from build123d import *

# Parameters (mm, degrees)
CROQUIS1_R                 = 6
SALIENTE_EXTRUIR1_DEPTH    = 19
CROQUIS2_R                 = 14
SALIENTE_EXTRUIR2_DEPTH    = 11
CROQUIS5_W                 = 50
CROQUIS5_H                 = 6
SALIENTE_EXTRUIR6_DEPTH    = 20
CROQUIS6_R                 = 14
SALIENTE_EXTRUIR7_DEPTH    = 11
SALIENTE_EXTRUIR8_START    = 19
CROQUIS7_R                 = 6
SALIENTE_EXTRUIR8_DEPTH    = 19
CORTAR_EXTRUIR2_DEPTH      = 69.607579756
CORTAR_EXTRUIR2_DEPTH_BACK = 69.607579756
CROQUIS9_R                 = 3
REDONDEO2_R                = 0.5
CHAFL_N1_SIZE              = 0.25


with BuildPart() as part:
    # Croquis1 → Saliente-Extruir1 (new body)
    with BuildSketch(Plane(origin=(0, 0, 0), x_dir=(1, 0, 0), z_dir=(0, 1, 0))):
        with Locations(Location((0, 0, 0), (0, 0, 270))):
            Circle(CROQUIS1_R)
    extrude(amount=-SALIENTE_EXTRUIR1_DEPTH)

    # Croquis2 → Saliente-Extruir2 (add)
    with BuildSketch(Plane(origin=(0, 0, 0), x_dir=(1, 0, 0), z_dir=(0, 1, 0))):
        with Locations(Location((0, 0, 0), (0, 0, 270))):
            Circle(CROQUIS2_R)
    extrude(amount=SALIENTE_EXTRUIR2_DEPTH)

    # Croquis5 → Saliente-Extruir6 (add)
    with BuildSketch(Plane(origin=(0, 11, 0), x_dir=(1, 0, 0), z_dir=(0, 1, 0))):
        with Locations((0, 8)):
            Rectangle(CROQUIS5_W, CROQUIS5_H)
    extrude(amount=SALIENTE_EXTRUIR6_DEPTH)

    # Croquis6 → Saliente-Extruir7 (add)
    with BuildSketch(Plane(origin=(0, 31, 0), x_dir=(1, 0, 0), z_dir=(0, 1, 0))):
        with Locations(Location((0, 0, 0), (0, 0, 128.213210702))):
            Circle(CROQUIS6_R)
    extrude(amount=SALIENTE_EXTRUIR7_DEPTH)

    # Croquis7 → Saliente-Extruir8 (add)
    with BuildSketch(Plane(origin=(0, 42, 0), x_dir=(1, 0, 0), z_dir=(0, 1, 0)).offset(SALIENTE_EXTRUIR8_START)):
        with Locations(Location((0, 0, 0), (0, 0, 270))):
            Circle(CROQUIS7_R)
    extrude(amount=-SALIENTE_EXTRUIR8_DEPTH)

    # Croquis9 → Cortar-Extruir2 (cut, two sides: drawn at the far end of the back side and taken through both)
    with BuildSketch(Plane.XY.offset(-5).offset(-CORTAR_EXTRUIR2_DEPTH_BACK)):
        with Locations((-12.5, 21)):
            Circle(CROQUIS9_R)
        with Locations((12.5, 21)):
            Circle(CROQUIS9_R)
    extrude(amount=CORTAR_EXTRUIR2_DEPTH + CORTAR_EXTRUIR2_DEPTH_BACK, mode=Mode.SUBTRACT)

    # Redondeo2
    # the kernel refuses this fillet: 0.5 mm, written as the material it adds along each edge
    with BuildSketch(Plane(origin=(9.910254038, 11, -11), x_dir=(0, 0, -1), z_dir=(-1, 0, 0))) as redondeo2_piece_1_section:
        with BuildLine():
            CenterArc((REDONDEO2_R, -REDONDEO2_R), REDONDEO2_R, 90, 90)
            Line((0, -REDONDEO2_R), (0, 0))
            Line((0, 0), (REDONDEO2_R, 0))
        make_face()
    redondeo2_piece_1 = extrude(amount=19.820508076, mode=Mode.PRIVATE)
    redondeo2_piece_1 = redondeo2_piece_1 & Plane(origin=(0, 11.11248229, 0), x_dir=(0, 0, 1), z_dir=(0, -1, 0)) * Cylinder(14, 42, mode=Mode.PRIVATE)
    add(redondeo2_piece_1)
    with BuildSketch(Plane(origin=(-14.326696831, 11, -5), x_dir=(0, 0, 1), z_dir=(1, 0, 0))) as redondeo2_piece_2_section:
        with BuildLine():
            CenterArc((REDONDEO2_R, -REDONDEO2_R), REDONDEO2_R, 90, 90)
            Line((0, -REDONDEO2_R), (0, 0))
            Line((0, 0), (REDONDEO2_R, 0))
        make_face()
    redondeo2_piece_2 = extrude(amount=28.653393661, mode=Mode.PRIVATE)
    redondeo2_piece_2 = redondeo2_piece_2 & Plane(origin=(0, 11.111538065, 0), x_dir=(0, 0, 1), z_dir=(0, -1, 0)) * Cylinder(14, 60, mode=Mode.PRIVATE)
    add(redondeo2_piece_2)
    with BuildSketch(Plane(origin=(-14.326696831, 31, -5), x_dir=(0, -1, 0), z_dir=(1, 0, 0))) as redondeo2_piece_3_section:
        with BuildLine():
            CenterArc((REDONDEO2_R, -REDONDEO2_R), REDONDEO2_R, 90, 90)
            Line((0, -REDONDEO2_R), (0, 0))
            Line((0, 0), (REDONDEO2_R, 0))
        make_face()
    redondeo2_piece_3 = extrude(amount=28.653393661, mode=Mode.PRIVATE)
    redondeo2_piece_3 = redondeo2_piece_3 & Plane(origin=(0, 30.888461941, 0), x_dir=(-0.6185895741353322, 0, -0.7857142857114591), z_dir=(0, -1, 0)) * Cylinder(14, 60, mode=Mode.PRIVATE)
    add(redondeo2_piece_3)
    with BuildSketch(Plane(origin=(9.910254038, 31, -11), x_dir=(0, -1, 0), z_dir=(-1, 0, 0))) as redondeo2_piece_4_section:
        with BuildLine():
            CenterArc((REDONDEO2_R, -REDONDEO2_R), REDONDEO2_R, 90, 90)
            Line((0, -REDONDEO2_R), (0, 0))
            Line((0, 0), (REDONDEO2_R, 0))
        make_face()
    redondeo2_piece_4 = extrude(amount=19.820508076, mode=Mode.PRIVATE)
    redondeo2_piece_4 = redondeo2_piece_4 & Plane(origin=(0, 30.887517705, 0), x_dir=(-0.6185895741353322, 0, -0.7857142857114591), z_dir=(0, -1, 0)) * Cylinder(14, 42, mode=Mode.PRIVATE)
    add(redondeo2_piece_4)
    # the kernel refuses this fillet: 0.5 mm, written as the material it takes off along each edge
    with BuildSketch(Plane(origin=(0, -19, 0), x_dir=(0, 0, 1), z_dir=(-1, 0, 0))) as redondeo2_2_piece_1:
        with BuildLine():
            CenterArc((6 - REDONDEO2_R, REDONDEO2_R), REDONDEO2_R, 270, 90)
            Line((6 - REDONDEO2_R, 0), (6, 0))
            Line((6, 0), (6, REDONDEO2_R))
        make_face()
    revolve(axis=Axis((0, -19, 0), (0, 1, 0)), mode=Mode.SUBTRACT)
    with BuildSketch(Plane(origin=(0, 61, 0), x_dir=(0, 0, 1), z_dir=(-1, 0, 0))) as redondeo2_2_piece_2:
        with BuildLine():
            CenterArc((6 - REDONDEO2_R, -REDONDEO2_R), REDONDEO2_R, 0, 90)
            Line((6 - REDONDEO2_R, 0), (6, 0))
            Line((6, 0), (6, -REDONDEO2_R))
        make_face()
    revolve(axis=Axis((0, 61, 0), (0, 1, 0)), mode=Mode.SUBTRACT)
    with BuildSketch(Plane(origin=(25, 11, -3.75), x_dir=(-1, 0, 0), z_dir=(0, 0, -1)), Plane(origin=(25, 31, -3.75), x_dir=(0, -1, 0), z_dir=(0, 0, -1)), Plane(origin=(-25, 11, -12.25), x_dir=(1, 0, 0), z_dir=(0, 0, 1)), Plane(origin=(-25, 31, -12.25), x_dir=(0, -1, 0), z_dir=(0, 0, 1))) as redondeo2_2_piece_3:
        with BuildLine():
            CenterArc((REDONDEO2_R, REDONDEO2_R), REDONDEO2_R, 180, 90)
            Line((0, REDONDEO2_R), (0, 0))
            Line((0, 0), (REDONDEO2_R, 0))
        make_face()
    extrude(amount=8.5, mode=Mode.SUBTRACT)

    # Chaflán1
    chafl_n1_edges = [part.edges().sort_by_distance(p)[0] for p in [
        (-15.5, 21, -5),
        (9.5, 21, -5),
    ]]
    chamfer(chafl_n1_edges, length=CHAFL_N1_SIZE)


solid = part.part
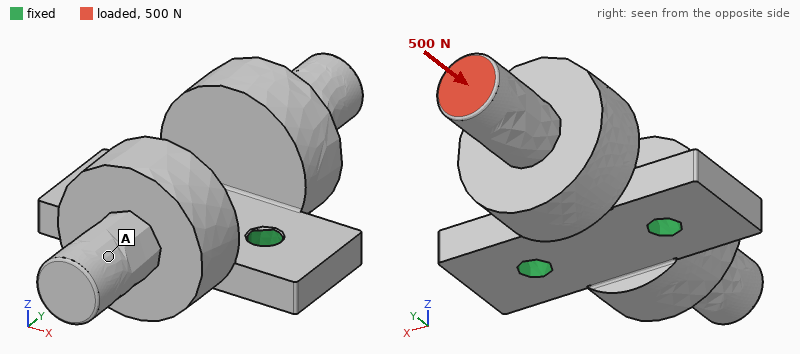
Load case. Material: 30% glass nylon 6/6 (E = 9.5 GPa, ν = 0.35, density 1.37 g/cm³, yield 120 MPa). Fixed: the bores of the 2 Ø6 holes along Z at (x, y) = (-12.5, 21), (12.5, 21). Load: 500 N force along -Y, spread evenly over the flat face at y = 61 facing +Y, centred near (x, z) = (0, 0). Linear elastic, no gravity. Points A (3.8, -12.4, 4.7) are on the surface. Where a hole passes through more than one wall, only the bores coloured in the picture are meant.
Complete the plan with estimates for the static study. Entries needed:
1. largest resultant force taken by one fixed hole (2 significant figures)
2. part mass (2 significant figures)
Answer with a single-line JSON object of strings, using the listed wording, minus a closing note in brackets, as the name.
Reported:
{"largest resultant force taken by one fixed hole": "260 N", "part mass": "32 g"}
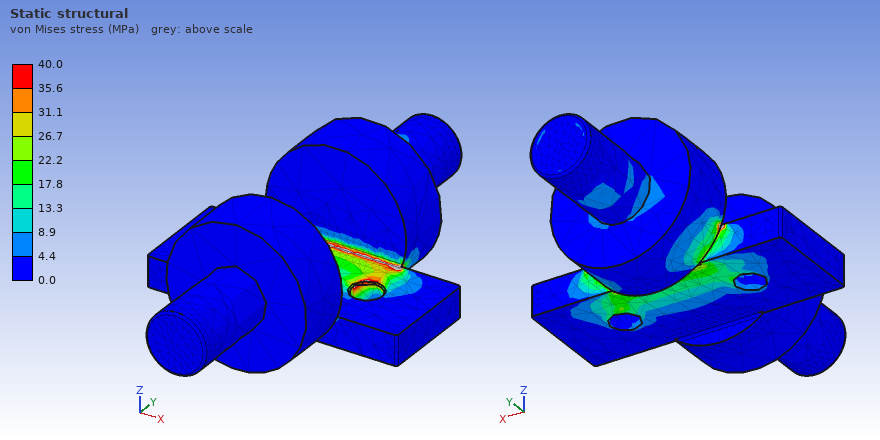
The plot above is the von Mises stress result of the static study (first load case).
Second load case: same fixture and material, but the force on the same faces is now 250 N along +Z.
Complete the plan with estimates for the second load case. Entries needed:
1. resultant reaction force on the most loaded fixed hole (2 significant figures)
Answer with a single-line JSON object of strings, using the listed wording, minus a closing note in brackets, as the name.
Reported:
{"resultant reaction force on the most loaded fixed hole": "130 N"}
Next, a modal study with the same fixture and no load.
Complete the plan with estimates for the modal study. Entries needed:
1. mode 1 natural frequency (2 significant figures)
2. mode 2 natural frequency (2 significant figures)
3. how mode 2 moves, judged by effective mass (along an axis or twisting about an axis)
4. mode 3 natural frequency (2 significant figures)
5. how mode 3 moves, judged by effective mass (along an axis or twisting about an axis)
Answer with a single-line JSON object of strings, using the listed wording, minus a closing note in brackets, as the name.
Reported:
{"mode 1 natural frequency": "1500 Hz", "mode 2 natural frequency": "1700 Hz", "how mode 2 moves, judged by effective mass": "along Z", "mode 3 natural frequency": "4900 Hz", "how mode 3 moves, judged by effective mass": "twisting about Z"}
